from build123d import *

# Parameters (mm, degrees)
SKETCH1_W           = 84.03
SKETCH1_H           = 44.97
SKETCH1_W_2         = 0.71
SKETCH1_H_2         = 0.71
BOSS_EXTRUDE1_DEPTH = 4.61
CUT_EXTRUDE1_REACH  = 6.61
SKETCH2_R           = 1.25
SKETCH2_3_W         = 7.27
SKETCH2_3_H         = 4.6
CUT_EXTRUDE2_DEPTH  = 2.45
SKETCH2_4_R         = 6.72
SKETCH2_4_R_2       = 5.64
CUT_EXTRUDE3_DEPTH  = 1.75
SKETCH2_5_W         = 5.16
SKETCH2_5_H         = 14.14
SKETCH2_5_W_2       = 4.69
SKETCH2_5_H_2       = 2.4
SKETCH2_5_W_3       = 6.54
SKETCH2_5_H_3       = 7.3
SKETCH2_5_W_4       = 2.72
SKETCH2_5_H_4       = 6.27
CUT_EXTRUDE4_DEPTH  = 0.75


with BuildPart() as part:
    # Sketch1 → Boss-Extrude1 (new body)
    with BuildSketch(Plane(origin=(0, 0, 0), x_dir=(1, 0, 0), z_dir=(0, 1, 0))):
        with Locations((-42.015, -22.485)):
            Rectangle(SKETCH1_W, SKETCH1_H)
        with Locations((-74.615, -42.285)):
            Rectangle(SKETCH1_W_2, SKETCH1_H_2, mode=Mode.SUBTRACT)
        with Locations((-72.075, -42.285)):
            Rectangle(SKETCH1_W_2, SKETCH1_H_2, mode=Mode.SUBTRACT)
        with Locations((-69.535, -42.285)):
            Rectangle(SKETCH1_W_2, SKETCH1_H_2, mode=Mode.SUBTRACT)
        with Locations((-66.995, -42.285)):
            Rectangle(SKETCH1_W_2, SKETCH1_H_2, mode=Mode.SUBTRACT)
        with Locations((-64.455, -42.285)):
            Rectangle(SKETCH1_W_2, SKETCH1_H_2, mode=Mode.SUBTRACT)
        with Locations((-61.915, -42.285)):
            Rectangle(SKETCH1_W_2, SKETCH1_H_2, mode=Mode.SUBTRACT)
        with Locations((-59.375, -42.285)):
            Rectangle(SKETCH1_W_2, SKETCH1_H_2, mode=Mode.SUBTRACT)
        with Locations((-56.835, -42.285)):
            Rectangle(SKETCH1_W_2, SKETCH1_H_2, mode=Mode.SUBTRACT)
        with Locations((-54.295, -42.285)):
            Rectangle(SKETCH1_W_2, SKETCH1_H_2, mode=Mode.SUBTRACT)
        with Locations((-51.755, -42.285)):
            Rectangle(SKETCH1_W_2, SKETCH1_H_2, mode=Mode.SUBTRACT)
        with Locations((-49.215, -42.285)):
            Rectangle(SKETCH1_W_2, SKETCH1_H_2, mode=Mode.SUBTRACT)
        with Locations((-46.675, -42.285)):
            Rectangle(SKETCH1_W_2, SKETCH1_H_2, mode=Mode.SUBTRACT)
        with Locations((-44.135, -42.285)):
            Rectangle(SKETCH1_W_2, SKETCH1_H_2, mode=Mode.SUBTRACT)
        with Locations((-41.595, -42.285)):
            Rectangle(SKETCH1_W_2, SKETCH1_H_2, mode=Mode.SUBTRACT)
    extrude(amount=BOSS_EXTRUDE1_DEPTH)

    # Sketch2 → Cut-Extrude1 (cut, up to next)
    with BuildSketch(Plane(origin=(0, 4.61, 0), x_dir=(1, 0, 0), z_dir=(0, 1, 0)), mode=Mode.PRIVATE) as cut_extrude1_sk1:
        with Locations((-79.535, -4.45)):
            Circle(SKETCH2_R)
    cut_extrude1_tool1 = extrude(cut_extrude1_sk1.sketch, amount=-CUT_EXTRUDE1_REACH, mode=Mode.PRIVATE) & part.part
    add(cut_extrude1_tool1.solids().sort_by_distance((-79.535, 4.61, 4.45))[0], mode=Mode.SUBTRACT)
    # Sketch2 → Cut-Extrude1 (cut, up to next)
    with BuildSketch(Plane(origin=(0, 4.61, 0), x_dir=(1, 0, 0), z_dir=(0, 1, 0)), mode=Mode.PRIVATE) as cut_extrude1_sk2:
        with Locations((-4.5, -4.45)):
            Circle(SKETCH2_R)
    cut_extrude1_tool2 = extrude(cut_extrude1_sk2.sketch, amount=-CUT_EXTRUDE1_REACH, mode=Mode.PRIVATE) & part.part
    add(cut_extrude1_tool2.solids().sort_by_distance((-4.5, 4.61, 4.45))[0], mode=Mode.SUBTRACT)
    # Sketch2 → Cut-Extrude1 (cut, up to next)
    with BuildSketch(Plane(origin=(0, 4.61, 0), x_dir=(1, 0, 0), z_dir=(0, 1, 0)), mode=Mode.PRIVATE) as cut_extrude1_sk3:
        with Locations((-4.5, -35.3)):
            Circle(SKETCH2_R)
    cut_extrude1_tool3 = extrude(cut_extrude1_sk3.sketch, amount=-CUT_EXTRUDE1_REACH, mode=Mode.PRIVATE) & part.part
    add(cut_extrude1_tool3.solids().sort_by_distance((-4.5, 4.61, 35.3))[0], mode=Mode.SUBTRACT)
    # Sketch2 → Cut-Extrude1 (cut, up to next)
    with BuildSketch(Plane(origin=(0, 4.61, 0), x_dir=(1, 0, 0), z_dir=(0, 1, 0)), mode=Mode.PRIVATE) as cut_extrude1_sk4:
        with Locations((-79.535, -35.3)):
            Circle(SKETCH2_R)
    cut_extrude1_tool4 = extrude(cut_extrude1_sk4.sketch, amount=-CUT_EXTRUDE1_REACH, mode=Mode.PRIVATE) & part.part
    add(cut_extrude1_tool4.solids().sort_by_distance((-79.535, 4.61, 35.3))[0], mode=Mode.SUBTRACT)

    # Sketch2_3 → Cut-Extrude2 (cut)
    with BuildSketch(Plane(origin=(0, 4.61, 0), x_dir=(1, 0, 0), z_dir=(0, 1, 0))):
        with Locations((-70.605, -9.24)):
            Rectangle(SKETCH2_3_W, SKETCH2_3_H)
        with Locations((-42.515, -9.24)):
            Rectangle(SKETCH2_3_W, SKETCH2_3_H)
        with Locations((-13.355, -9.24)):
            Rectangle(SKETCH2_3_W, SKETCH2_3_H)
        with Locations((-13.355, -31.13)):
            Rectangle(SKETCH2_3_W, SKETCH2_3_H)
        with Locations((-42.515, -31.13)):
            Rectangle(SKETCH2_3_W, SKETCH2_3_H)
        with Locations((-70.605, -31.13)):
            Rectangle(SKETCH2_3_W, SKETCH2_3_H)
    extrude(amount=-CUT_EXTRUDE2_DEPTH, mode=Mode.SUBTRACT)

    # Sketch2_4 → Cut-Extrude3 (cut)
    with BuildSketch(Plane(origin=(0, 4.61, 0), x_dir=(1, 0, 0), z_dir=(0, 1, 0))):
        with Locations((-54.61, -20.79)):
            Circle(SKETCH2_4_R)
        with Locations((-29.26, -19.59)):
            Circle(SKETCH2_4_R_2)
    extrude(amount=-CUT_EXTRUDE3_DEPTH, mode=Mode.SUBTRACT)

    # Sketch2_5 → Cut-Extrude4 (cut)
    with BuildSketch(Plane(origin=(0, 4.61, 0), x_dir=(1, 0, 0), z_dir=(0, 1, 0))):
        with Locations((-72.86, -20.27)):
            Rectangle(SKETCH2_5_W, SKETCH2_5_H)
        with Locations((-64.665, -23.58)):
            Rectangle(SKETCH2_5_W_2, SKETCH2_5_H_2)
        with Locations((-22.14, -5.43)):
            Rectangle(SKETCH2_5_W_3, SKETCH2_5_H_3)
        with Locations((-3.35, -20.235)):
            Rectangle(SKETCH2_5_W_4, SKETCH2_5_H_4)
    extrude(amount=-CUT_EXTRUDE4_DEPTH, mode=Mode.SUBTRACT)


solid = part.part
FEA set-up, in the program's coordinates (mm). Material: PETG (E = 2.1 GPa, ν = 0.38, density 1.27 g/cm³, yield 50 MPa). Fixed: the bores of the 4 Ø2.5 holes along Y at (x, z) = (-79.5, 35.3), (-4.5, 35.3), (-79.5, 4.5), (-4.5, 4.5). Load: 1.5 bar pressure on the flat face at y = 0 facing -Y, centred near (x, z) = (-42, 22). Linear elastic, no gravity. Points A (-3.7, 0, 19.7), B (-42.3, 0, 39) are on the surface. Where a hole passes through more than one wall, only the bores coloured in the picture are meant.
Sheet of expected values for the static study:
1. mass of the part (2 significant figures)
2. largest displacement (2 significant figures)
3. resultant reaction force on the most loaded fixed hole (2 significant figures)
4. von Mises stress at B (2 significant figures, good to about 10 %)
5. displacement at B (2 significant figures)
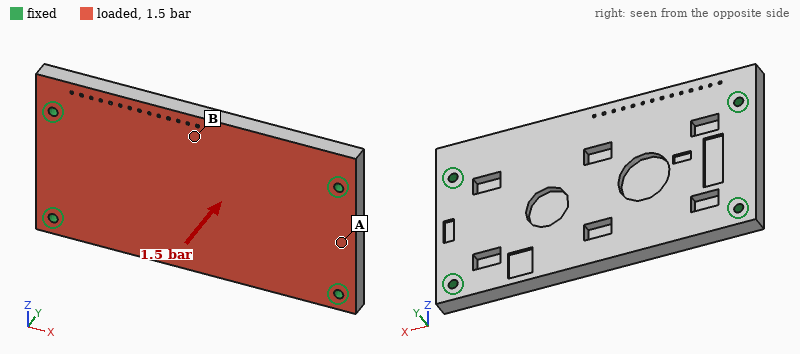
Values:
21 g
1.1 mm
160 N
13 MPa
1.1 mm
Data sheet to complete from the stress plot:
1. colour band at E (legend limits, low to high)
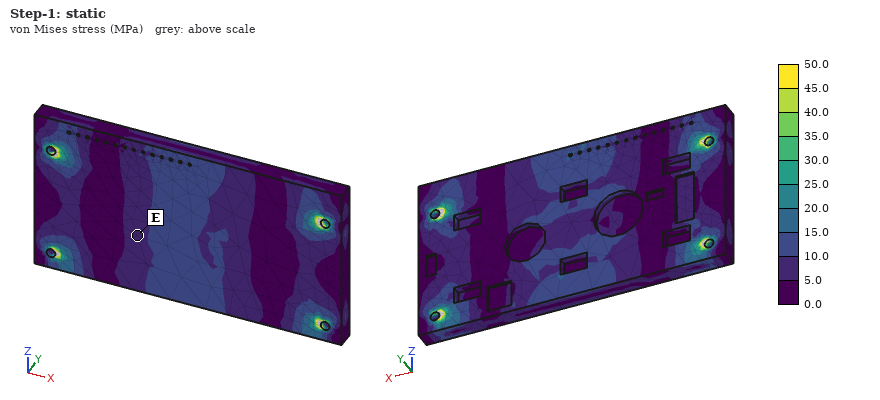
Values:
5.0 to 10.0 MPa
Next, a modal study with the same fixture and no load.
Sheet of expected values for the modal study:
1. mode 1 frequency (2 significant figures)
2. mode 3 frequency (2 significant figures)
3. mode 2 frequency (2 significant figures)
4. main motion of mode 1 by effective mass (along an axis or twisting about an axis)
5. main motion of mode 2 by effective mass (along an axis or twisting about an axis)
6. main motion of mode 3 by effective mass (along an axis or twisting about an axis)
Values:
910 Hz
2500 Hz
1400 Hz
along Y
twisting about X
twisting about Z
